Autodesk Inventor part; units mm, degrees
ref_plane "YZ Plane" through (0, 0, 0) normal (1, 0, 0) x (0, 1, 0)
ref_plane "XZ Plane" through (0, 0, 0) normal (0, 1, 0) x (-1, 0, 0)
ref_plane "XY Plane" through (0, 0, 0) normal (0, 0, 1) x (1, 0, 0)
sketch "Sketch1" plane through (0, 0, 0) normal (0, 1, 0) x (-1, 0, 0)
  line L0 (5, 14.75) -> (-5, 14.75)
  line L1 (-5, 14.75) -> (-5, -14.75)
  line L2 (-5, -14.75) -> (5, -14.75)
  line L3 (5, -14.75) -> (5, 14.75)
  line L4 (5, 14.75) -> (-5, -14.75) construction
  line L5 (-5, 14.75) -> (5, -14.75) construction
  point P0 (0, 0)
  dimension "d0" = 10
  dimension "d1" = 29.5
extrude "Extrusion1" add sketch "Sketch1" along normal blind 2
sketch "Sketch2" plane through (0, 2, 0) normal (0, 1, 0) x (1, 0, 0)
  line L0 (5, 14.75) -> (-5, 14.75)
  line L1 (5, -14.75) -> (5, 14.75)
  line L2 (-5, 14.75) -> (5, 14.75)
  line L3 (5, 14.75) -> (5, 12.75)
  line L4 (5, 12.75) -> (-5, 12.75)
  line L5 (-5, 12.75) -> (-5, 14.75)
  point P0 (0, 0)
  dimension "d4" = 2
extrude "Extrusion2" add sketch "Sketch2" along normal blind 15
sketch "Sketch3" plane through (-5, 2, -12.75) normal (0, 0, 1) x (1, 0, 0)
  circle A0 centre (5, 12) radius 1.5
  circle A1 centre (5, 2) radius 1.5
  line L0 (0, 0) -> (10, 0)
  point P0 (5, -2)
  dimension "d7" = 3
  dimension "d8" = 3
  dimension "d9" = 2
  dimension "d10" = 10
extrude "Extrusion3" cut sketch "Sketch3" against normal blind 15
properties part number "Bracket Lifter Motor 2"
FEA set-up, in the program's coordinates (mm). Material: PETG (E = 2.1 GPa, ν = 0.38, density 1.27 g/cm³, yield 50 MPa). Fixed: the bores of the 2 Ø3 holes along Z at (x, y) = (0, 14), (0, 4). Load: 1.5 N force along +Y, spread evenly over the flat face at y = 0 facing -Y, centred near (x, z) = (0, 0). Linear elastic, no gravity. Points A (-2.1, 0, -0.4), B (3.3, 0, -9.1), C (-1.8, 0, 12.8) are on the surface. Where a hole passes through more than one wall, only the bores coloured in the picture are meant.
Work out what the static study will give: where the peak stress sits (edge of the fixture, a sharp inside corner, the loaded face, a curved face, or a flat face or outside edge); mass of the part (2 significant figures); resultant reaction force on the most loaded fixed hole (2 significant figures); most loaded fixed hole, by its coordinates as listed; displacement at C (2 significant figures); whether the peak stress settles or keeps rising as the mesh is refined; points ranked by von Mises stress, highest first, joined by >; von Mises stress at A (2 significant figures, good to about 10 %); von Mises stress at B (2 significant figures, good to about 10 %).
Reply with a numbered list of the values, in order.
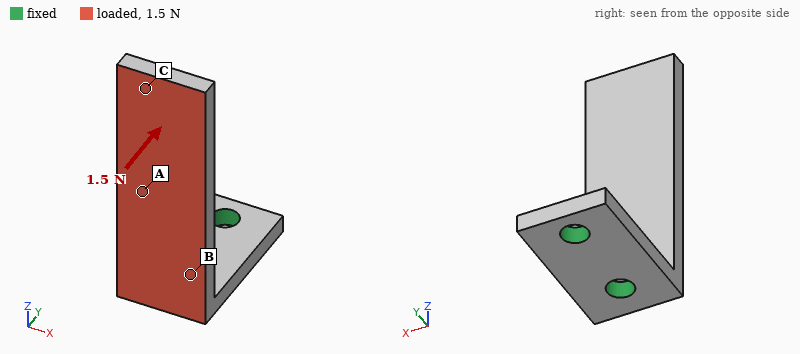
1. edge of the fixture
2. 1.1 g
3. 1.7 N
4. (0, 4)
5. 0.33 mm
6. keeps rising
7. B > A > C
8. 0.89 MPa
9. 2.1 MPa
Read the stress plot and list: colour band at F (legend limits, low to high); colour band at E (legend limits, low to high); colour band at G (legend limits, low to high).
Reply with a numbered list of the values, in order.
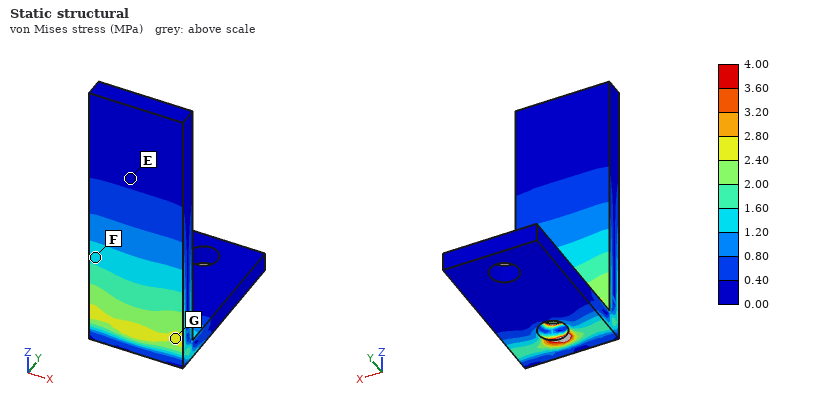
1. 1.20 to 1.60 MPa
2. 0.00 to 0.40 MPa
3. 2.40 to 2.80 MPa
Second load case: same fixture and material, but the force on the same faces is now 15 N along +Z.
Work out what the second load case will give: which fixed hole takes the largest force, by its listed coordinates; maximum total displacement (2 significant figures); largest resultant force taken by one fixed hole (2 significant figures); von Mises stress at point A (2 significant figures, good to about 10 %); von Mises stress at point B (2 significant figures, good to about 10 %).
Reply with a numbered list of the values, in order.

1. (0, 4)
2. 0.42 mm
3. 16 N
4. 1.5 MPa
5. 2.3 MPa
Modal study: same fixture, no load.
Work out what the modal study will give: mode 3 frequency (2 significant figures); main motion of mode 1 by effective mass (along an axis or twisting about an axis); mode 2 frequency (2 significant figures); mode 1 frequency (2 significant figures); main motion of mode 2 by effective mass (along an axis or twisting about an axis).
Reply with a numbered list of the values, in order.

1. 2700 Hz
2. along Y
3. 1100 Hz
4. 470 Hz
5. along X
